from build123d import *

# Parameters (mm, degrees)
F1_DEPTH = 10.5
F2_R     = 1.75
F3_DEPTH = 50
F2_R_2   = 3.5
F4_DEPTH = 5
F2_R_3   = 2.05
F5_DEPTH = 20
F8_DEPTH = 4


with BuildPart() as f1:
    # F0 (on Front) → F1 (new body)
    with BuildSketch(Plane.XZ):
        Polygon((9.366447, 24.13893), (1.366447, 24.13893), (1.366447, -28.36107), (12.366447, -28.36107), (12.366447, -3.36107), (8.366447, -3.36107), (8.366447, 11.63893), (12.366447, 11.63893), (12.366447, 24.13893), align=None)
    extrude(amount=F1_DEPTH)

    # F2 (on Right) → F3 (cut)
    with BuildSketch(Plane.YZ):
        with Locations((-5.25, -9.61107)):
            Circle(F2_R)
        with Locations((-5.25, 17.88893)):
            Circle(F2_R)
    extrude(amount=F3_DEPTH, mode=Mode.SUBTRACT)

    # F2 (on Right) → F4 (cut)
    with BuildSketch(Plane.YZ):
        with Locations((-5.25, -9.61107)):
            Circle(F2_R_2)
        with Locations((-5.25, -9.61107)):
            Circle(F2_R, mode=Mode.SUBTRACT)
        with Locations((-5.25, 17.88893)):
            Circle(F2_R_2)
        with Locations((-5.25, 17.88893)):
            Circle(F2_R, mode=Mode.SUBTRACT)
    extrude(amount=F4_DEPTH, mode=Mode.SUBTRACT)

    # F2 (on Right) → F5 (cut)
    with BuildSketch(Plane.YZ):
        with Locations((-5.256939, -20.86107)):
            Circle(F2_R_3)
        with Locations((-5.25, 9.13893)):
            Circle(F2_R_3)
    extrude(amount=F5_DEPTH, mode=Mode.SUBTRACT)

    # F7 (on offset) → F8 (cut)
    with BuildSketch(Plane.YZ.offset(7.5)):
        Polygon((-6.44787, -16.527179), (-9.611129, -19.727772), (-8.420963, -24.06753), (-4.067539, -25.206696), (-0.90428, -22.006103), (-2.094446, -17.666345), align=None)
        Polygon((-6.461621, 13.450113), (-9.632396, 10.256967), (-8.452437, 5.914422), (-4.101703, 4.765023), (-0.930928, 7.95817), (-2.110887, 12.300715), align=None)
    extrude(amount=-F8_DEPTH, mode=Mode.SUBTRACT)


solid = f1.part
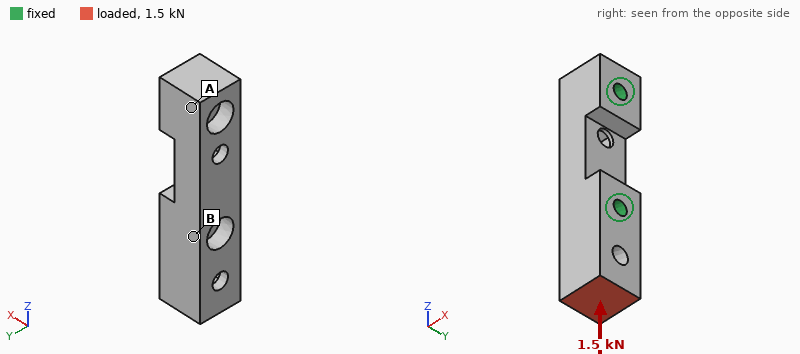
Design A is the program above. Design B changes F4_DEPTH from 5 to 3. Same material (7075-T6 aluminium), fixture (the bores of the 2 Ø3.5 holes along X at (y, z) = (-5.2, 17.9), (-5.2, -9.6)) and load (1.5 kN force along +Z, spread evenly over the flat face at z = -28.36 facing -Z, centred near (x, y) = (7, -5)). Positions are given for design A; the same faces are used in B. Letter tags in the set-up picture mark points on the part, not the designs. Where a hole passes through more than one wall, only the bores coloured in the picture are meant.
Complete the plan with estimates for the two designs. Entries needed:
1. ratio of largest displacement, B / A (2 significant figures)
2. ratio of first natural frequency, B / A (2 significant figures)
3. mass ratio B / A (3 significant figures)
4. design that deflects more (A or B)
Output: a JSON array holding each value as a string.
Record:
["0.71", "1.1", "1.03", "A"]
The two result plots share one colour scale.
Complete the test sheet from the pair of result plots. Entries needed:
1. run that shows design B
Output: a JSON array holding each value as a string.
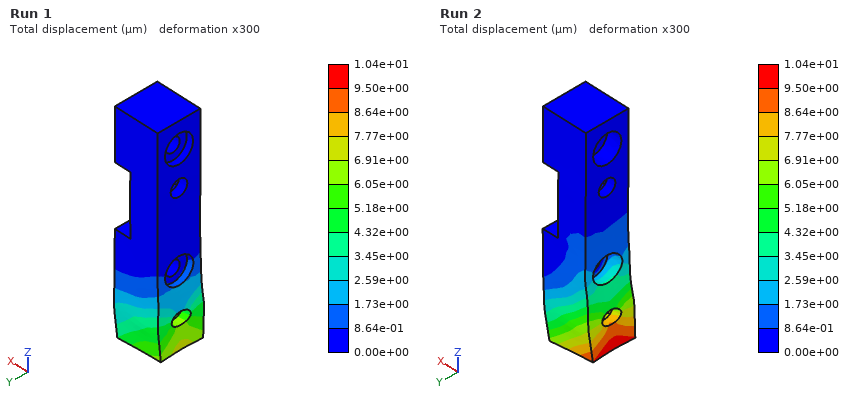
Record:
["Run 1"]
